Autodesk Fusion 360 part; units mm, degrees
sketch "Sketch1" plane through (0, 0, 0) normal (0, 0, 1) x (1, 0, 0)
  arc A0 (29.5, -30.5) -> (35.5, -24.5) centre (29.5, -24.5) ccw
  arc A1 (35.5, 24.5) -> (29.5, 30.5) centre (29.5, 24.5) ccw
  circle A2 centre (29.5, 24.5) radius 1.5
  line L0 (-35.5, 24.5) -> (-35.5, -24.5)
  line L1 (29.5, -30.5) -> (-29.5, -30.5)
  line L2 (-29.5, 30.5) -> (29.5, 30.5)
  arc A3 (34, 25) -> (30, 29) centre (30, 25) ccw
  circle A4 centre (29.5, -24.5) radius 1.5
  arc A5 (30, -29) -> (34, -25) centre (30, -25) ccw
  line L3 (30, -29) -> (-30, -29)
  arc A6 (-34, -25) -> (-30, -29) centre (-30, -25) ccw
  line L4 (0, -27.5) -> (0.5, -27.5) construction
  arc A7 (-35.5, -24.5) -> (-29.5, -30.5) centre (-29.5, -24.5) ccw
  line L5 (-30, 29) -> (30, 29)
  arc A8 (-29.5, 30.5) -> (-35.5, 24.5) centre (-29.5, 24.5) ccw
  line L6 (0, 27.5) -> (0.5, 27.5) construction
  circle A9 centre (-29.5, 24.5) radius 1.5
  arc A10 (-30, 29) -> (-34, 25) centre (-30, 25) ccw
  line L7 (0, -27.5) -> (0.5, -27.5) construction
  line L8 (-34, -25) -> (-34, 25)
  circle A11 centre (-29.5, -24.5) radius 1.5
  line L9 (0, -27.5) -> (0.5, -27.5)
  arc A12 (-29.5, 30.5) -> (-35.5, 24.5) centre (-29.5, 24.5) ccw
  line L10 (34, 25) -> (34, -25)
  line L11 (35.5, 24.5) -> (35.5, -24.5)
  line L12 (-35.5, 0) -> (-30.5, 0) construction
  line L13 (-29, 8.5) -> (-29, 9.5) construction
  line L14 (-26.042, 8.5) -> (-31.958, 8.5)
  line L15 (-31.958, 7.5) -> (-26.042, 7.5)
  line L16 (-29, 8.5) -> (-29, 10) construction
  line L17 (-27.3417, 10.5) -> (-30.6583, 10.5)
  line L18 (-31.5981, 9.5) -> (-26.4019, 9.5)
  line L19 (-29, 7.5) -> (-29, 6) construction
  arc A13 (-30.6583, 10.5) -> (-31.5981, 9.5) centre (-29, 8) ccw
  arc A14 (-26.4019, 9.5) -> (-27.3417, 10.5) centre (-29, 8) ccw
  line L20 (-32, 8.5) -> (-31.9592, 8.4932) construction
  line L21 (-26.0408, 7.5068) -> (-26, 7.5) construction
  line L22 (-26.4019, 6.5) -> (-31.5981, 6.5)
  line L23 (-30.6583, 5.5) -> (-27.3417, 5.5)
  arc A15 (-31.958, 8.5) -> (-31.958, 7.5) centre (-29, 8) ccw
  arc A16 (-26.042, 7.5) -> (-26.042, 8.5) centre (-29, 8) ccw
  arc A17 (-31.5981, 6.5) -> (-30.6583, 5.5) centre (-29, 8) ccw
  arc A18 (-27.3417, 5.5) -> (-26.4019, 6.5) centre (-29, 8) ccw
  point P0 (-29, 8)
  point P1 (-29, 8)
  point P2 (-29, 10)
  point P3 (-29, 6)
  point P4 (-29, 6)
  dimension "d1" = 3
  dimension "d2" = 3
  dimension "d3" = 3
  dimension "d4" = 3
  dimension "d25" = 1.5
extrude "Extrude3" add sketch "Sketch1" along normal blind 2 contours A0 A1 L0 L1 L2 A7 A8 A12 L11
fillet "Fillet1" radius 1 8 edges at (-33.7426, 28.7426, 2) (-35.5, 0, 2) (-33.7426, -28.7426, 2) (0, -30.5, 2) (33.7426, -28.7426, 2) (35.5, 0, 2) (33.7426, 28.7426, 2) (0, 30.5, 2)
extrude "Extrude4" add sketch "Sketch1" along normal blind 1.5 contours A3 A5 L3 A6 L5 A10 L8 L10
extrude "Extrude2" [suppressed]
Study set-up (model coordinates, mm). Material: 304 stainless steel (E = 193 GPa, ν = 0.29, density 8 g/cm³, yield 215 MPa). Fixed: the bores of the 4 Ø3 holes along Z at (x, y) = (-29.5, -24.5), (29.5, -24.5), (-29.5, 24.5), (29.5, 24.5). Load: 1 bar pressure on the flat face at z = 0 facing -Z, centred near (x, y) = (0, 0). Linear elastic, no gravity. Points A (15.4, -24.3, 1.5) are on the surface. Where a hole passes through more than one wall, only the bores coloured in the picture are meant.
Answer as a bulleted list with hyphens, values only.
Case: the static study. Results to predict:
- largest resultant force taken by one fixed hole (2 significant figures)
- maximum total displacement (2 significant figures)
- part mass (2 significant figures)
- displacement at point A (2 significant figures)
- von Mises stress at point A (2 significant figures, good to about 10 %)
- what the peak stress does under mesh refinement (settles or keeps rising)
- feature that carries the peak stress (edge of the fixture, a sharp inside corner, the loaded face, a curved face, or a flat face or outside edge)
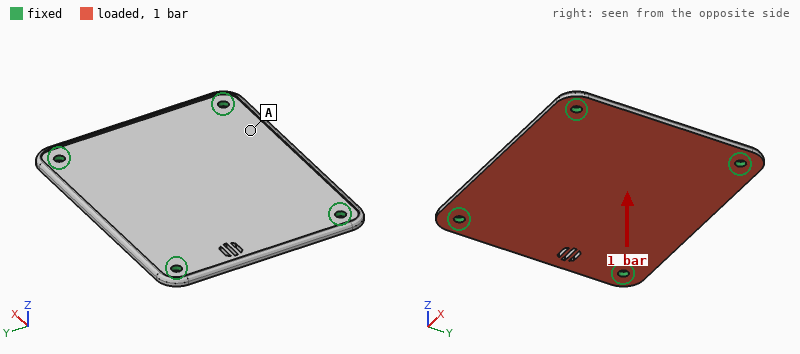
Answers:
- 110 N
- 0.10 mm
- 52 g
- 0.039 mm
- 17 MPa
- keeps rising
- edge of the fixture
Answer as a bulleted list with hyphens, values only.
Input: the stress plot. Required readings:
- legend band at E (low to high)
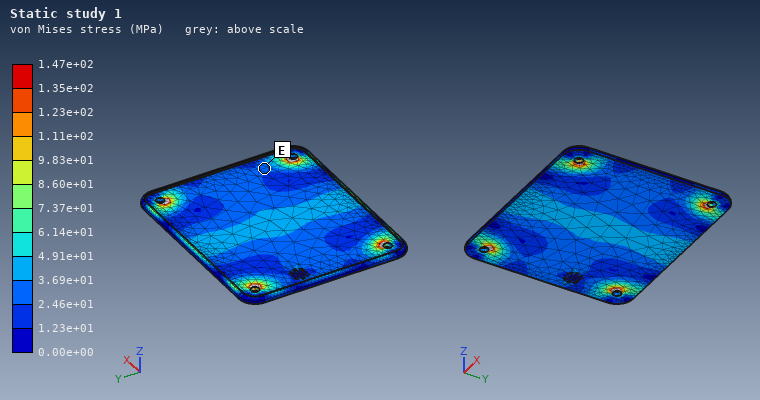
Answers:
- 2.46e+01 to 3.69e+01 MPa
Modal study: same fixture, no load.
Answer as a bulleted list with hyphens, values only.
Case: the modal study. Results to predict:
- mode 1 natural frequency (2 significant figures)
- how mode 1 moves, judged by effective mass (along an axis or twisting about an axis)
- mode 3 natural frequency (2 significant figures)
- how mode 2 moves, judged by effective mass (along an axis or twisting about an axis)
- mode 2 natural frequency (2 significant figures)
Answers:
- 1700 Hz
- along Z
- 3300 Hz
- twisting about X
- 2700 Hz
